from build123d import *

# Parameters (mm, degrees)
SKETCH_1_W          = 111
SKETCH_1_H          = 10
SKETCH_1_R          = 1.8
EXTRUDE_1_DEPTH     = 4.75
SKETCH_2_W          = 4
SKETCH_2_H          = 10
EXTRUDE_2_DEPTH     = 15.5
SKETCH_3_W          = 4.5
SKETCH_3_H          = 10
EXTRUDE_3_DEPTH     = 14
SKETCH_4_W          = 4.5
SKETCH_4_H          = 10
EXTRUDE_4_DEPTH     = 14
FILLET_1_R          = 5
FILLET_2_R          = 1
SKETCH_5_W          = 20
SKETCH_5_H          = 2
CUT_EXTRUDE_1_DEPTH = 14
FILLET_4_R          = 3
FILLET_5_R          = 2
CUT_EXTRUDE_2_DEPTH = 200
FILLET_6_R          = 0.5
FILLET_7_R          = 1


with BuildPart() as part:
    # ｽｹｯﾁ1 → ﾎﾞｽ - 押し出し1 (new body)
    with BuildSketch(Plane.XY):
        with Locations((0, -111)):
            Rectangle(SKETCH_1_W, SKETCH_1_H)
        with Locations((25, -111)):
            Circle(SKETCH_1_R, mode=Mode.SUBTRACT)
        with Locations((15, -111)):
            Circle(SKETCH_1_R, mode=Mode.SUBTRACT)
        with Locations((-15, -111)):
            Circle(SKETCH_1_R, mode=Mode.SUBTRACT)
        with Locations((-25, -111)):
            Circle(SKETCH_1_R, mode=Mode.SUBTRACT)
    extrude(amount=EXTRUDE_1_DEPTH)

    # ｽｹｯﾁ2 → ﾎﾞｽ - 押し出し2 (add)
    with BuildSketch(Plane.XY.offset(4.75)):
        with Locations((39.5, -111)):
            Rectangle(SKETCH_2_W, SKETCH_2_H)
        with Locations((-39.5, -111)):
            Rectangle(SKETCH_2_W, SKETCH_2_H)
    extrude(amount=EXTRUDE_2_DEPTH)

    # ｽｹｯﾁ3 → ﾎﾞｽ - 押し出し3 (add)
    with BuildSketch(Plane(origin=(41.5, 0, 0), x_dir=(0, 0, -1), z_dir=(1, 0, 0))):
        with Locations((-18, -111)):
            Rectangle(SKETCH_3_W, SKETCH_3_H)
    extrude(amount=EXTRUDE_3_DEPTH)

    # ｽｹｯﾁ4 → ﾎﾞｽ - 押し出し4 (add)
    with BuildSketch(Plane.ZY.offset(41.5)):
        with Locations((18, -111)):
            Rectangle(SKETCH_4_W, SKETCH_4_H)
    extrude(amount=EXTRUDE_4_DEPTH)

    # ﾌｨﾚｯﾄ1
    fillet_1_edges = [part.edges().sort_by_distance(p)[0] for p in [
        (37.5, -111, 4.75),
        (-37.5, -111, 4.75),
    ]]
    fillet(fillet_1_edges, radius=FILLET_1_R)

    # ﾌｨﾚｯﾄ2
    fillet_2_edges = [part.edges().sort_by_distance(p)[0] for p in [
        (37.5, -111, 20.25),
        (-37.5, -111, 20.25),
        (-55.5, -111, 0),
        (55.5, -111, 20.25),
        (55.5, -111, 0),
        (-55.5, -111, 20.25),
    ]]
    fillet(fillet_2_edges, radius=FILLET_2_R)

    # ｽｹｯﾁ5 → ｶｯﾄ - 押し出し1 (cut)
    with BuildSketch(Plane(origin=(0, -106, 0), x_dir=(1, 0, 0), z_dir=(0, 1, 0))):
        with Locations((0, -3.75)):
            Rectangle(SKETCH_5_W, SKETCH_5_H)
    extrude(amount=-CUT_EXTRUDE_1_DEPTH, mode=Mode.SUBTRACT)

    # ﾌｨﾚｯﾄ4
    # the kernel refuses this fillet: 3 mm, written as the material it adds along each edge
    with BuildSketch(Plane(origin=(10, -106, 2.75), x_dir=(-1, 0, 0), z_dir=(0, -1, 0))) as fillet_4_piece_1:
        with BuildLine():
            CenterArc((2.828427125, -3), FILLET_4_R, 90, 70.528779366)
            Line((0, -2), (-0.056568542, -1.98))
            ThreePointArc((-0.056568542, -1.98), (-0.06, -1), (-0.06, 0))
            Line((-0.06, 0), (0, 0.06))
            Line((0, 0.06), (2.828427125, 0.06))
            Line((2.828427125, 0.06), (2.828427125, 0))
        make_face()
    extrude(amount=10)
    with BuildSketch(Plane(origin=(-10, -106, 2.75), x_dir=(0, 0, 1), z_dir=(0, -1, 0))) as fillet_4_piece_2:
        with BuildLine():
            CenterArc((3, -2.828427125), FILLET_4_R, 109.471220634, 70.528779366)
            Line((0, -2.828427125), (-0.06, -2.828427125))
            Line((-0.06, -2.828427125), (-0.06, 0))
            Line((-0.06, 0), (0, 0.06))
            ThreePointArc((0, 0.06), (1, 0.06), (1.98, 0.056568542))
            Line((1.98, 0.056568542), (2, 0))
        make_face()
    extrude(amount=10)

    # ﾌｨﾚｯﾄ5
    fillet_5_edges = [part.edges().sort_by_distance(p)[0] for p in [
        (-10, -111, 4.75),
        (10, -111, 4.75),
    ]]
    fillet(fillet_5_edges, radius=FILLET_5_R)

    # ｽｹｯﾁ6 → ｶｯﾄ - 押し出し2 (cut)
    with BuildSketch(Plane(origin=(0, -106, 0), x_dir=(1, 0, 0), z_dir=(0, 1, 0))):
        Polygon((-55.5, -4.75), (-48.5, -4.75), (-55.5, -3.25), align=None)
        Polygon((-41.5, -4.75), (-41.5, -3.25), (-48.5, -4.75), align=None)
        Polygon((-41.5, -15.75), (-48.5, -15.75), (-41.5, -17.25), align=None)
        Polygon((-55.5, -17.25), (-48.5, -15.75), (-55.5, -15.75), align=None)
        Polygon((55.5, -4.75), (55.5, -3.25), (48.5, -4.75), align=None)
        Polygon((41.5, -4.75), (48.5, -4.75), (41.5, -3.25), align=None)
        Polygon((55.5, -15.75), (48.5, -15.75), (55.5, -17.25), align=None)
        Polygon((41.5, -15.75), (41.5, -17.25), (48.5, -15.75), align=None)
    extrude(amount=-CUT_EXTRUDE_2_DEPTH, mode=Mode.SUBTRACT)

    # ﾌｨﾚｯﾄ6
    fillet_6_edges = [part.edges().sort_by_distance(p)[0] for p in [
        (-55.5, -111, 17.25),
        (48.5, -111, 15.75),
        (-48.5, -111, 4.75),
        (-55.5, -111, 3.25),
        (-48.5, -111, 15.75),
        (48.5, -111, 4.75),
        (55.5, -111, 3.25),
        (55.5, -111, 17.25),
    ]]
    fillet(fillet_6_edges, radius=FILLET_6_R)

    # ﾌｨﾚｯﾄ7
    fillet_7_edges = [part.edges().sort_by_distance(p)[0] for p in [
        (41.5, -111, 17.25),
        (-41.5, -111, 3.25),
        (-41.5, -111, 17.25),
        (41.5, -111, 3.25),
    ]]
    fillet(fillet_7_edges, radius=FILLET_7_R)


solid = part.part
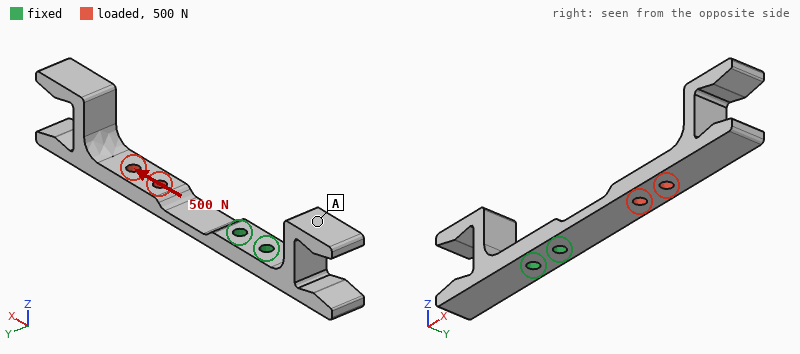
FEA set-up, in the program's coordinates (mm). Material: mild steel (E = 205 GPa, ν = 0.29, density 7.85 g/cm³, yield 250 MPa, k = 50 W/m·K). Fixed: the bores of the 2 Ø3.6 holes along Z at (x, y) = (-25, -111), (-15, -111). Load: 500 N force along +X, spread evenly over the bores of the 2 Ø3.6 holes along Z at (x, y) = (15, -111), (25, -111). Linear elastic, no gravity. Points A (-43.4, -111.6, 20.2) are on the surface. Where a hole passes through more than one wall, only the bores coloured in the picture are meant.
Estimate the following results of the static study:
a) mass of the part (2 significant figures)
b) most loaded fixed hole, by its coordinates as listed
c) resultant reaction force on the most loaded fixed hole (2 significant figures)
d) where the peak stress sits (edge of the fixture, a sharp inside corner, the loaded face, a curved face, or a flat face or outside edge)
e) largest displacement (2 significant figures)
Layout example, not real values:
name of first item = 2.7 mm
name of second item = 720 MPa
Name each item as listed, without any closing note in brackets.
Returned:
mass of the part = 54 g
most loaded fixed hole, by its coordinates as listed = (-15, -111)
resultant reaction force on the most loaded fixed hole = 450 N
where the peak stress sits = a curved face
largest displacement = 0.15 mm
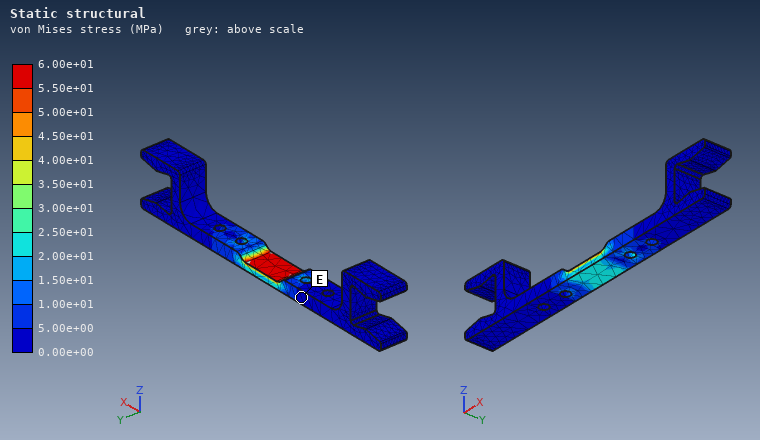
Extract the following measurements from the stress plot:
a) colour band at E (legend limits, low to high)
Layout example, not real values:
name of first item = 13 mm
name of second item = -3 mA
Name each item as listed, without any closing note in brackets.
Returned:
colour band at E = 0.00e+00 to 5.00e+00 MPa
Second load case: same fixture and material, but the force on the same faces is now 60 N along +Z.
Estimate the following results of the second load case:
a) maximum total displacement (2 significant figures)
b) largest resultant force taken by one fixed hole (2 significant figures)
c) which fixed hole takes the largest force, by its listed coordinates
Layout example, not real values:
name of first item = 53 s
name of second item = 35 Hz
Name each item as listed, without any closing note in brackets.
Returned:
maximum total displacement = 0.42 mm
largest resultant force taken by one fixed hole = 88 N
which fixed hole takes the largest force, by its listed coordinates = (-15, -111)
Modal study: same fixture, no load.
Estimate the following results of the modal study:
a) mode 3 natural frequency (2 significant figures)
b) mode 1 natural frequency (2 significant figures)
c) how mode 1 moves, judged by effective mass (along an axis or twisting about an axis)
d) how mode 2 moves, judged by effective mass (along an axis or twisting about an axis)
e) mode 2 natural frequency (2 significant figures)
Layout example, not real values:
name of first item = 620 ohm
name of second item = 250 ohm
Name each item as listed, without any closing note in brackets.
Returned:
mode 3 natural frequency = 2200 Hz
mode 1 natural frequency = 330 Hz
how mode 1 moves, judged by effective mass = along Z
how mode 2 moves, judged by effective mass = along Y
mode 2 natural frequency = 890 Hz
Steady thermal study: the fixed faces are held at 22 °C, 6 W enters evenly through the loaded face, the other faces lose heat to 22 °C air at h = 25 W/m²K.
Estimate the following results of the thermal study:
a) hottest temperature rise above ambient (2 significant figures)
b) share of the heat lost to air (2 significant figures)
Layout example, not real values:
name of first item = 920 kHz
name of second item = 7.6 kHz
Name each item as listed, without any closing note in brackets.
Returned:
hottest temperature rise above ambient = 62 K
share of the heat lost to air = 51 %
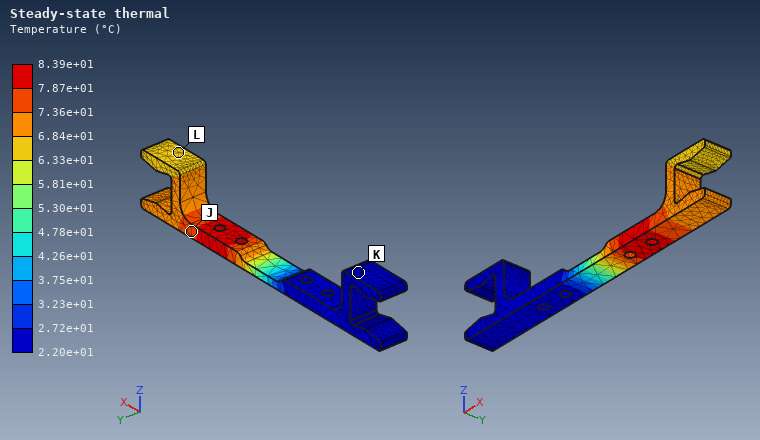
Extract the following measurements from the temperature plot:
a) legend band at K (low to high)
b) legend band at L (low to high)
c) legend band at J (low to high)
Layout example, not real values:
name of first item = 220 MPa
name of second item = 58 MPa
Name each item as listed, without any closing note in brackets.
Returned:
legend band at K = 2.20e+01 to 2.72e+01 °C
legend band at L = 6.33e+01 to 6.84e+01 °C
legend band at J = 7.36e+01 to 7.87e+01 °C
